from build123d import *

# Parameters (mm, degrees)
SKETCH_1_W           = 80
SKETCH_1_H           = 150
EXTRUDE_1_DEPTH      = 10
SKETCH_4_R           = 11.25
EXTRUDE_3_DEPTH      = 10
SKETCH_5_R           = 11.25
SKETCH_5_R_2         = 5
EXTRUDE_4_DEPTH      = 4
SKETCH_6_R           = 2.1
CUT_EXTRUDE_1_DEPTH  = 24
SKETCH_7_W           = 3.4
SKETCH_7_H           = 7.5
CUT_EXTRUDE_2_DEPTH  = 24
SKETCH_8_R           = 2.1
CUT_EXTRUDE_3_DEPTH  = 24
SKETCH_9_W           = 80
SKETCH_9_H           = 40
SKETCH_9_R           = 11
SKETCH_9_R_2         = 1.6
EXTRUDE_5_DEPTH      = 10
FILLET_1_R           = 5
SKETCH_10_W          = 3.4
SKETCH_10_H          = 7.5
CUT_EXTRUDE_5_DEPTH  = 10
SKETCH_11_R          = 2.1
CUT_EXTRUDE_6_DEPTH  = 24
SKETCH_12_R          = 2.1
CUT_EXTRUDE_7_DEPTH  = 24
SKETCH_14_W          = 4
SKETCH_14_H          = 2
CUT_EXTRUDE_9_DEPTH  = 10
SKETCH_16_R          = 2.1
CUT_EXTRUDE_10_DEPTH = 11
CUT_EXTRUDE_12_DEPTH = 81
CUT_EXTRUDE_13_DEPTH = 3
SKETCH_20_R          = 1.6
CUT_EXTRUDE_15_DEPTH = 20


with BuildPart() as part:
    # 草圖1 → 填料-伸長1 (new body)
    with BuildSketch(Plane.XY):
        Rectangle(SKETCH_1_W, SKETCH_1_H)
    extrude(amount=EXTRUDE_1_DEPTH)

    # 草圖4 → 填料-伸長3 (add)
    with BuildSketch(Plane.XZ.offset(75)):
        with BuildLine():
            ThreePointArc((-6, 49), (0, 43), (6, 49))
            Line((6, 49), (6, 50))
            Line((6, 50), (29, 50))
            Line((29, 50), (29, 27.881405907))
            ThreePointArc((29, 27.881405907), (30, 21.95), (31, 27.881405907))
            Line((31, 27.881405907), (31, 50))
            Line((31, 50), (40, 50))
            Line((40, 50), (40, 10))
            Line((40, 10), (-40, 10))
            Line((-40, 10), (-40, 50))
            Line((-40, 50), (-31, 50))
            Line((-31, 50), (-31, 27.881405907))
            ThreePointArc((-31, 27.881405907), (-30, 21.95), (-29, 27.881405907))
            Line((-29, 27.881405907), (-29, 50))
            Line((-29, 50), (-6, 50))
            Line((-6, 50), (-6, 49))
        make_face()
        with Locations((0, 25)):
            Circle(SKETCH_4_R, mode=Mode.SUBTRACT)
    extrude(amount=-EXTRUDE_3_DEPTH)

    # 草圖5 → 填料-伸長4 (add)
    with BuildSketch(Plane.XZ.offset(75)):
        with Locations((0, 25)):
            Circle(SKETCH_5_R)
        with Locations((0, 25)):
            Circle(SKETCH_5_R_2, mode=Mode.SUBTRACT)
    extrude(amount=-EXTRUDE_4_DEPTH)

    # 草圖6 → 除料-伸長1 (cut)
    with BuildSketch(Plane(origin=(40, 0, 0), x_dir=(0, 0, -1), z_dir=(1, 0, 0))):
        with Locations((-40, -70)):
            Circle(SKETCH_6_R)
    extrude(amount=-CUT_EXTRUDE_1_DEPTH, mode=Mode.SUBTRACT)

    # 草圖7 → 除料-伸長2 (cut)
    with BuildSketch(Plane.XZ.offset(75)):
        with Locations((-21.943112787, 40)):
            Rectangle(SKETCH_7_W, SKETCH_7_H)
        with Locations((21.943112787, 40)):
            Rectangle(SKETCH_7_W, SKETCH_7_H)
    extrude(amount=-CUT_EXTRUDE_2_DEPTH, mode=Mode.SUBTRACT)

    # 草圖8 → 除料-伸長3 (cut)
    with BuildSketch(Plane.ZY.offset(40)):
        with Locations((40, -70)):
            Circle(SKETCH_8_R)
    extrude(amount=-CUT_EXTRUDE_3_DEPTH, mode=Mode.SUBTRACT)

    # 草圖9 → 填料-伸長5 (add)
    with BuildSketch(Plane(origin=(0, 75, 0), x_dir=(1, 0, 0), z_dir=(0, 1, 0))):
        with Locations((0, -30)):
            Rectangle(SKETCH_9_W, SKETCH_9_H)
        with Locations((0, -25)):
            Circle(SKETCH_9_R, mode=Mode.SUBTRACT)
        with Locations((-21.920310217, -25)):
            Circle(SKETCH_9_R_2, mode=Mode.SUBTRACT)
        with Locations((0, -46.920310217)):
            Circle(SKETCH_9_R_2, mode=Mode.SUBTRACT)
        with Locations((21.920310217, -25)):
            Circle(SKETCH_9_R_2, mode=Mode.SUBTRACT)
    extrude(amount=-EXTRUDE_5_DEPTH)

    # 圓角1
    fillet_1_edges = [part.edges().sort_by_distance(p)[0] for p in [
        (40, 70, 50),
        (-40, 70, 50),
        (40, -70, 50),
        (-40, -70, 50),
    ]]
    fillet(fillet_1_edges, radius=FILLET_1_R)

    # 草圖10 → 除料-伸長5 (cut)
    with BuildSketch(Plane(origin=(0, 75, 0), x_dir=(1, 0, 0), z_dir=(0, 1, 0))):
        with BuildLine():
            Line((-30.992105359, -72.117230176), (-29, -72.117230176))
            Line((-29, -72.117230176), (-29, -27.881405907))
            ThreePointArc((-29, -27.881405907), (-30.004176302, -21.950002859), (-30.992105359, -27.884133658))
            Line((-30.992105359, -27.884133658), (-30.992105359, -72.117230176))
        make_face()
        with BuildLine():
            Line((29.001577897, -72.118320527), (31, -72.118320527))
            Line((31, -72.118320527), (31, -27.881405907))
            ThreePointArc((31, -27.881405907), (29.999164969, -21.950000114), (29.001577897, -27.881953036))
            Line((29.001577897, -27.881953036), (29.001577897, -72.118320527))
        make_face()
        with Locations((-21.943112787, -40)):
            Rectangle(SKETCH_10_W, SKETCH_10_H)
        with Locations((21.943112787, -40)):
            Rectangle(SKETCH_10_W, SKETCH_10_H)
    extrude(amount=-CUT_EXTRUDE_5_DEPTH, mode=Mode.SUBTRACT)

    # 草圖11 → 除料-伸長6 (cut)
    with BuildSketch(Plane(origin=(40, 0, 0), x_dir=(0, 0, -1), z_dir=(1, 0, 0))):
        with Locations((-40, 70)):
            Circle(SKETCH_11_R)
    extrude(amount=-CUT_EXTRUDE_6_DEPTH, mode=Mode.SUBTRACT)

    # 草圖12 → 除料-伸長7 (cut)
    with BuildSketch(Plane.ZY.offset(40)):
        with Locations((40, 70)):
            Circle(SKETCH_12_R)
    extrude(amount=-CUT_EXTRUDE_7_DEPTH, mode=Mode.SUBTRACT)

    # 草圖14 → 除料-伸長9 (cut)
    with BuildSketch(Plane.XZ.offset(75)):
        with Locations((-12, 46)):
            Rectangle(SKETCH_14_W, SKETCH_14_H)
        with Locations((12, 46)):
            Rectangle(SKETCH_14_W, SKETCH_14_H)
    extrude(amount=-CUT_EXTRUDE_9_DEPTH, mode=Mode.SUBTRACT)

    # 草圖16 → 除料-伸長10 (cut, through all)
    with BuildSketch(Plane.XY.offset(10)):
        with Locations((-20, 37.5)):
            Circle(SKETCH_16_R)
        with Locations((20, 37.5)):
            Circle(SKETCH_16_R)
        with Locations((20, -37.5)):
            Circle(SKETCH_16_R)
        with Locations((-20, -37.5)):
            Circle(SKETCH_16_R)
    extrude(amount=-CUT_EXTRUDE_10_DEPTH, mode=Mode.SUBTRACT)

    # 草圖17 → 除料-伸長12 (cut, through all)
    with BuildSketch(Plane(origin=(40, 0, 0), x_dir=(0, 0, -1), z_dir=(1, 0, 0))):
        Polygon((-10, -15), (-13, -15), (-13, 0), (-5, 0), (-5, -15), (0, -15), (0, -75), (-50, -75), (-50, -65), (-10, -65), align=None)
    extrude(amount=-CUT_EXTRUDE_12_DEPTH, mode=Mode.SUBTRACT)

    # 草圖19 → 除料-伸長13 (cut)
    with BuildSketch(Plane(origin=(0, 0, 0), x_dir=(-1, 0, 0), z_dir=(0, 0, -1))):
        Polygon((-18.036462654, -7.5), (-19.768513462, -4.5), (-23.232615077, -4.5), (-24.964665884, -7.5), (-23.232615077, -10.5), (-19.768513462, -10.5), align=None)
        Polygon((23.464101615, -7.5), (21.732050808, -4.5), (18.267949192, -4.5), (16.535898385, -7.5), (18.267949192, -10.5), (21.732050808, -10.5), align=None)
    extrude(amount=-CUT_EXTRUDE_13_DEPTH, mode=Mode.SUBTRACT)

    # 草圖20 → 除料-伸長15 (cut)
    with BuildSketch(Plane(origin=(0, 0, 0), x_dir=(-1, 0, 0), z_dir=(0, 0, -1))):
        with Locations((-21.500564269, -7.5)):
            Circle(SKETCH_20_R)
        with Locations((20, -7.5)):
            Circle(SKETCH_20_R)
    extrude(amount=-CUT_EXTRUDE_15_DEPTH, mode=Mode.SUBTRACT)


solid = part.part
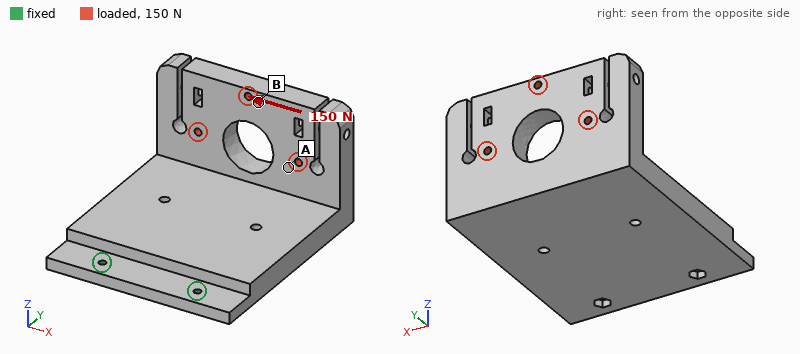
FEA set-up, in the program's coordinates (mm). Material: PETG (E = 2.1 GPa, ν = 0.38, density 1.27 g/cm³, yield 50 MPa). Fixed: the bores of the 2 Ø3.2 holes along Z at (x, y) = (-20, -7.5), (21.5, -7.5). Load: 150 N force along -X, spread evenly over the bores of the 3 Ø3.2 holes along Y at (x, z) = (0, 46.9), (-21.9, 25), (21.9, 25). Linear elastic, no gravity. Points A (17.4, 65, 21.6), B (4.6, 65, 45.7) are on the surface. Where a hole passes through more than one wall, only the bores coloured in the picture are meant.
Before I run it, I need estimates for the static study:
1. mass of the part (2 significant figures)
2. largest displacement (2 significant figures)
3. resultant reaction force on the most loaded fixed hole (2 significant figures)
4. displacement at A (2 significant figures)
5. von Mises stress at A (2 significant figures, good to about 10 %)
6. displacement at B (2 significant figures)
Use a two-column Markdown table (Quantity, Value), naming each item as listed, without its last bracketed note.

| Quantity | Value |
|---|---|
| mass of the part | 120 g |
| largest displacement | 1.4 mm |
| resultant reaction force on the most loaded fixed hole | 300 N |
| displacement at A | 0.63 mm |
| von Mises stress at A | 1.8 MPa |
| displacement at B | 1.0 mm |
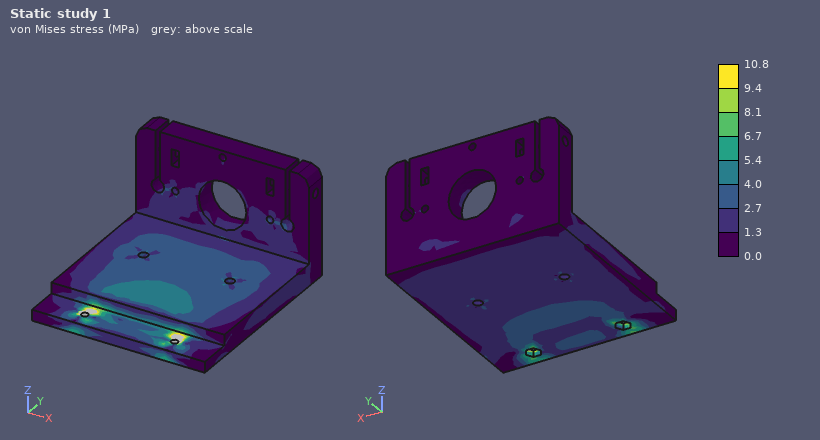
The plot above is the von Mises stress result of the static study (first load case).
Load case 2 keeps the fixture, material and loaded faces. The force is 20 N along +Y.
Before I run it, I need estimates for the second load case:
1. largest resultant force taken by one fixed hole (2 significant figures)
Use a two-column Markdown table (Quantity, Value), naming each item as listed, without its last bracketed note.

| Quantity | Value |
|---|---|
| largest resultant force taken by one fixed hole | 10 N |
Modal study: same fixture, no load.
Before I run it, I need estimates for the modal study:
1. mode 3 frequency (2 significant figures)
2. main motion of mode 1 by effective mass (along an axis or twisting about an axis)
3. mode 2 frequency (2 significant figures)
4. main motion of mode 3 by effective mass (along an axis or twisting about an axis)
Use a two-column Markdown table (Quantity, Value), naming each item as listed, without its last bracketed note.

| Quantity | Value |
|---|---|
| mode 3 frequency | 560 Hz |
| main motion of mode 1 by effective mass | along Z |
| mode 2 frequency | 270 Hz |
| main motion of mode 3 by effective mass | along X |
